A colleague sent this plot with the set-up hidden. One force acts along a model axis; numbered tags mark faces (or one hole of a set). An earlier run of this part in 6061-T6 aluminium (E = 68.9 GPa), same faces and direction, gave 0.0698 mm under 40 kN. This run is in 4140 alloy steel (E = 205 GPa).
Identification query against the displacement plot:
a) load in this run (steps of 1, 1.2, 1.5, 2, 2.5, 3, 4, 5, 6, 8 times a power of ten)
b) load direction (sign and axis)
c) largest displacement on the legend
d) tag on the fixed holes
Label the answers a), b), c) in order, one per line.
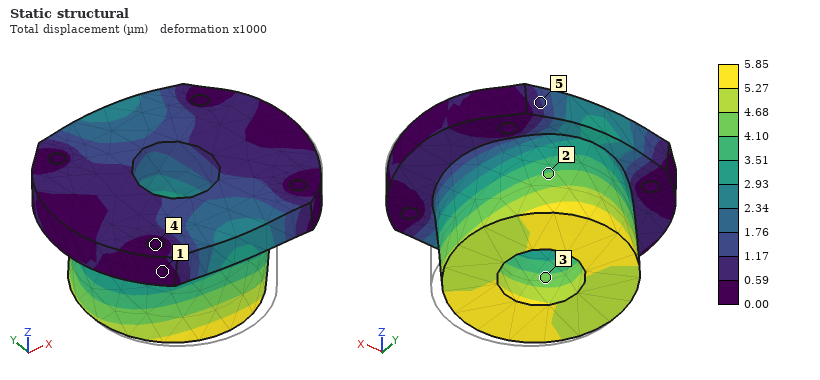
a) 10 kN
b) +Y
c) 5.85 µm
d) 4
